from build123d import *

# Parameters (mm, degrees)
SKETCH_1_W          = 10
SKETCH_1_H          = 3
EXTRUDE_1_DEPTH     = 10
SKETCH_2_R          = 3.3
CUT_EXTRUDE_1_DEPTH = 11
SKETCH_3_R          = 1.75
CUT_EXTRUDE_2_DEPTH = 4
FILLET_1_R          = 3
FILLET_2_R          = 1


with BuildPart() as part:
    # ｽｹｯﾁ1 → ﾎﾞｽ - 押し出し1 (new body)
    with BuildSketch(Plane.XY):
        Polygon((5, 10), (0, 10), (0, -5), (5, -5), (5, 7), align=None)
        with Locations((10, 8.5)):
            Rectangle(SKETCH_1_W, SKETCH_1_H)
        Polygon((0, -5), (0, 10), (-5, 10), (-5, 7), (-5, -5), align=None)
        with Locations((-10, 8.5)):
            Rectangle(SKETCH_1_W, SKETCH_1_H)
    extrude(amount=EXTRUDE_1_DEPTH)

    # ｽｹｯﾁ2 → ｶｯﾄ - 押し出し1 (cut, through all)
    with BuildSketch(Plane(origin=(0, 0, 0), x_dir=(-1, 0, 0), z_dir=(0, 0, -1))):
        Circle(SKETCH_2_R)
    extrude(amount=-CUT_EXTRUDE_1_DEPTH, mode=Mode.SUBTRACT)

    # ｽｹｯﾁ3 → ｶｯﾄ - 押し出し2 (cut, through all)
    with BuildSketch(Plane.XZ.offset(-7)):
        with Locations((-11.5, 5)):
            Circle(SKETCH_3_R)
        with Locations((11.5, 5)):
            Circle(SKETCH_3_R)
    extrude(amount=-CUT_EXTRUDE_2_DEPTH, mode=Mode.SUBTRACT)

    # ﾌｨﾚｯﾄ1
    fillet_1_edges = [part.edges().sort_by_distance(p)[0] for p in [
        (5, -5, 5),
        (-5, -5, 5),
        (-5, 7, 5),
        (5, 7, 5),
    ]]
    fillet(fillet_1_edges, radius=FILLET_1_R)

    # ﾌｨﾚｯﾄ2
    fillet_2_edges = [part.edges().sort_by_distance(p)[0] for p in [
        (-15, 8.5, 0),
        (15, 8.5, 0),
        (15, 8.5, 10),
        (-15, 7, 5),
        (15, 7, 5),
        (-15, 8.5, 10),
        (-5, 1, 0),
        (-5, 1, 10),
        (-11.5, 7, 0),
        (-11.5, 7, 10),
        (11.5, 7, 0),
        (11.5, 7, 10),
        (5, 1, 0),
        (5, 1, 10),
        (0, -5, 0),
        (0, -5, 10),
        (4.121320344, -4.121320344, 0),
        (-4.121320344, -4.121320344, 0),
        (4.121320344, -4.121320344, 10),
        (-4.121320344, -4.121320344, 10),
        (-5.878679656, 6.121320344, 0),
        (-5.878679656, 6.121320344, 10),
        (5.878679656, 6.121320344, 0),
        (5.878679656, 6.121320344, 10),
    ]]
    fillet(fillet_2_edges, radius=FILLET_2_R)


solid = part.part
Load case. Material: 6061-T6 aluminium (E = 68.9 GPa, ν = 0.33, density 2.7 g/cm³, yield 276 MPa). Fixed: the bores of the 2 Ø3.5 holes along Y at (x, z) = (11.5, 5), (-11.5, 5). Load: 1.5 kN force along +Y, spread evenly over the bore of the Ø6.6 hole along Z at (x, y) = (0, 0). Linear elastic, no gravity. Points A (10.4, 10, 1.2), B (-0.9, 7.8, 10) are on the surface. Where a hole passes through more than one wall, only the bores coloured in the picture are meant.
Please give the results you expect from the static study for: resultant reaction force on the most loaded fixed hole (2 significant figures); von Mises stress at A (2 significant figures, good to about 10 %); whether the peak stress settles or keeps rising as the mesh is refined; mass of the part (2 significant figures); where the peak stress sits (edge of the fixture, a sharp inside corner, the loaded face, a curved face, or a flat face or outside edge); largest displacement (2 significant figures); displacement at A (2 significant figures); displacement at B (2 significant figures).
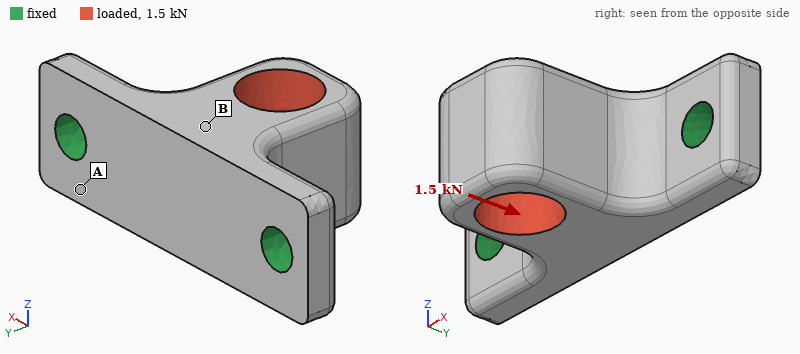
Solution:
850 N
50 MPa
keeps rising
4.5 g
edge of the fixture
22 µm
3.7 µm
17 µm
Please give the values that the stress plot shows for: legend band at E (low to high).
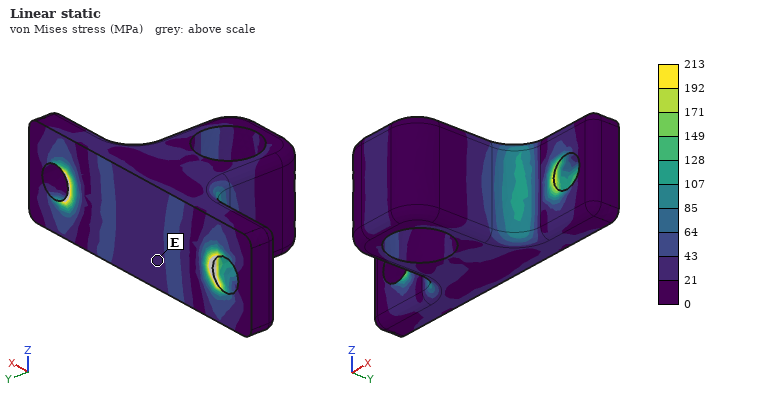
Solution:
21 to 43 MPa
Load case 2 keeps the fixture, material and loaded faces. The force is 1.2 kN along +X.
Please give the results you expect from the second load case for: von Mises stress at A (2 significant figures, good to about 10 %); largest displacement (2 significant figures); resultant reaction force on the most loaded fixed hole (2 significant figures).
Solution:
27 MPa
43 µm
840 N
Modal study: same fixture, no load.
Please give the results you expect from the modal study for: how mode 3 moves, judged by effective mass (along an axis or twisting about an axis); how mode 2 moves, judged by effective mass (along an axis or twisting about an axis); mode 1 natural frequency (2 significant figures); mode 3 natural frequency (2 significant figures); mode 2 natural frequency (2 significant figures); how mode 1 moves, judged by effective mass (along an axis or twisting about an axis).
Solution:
along Y
along X
12 kHz
26 kHz
24 kHz
along Z
